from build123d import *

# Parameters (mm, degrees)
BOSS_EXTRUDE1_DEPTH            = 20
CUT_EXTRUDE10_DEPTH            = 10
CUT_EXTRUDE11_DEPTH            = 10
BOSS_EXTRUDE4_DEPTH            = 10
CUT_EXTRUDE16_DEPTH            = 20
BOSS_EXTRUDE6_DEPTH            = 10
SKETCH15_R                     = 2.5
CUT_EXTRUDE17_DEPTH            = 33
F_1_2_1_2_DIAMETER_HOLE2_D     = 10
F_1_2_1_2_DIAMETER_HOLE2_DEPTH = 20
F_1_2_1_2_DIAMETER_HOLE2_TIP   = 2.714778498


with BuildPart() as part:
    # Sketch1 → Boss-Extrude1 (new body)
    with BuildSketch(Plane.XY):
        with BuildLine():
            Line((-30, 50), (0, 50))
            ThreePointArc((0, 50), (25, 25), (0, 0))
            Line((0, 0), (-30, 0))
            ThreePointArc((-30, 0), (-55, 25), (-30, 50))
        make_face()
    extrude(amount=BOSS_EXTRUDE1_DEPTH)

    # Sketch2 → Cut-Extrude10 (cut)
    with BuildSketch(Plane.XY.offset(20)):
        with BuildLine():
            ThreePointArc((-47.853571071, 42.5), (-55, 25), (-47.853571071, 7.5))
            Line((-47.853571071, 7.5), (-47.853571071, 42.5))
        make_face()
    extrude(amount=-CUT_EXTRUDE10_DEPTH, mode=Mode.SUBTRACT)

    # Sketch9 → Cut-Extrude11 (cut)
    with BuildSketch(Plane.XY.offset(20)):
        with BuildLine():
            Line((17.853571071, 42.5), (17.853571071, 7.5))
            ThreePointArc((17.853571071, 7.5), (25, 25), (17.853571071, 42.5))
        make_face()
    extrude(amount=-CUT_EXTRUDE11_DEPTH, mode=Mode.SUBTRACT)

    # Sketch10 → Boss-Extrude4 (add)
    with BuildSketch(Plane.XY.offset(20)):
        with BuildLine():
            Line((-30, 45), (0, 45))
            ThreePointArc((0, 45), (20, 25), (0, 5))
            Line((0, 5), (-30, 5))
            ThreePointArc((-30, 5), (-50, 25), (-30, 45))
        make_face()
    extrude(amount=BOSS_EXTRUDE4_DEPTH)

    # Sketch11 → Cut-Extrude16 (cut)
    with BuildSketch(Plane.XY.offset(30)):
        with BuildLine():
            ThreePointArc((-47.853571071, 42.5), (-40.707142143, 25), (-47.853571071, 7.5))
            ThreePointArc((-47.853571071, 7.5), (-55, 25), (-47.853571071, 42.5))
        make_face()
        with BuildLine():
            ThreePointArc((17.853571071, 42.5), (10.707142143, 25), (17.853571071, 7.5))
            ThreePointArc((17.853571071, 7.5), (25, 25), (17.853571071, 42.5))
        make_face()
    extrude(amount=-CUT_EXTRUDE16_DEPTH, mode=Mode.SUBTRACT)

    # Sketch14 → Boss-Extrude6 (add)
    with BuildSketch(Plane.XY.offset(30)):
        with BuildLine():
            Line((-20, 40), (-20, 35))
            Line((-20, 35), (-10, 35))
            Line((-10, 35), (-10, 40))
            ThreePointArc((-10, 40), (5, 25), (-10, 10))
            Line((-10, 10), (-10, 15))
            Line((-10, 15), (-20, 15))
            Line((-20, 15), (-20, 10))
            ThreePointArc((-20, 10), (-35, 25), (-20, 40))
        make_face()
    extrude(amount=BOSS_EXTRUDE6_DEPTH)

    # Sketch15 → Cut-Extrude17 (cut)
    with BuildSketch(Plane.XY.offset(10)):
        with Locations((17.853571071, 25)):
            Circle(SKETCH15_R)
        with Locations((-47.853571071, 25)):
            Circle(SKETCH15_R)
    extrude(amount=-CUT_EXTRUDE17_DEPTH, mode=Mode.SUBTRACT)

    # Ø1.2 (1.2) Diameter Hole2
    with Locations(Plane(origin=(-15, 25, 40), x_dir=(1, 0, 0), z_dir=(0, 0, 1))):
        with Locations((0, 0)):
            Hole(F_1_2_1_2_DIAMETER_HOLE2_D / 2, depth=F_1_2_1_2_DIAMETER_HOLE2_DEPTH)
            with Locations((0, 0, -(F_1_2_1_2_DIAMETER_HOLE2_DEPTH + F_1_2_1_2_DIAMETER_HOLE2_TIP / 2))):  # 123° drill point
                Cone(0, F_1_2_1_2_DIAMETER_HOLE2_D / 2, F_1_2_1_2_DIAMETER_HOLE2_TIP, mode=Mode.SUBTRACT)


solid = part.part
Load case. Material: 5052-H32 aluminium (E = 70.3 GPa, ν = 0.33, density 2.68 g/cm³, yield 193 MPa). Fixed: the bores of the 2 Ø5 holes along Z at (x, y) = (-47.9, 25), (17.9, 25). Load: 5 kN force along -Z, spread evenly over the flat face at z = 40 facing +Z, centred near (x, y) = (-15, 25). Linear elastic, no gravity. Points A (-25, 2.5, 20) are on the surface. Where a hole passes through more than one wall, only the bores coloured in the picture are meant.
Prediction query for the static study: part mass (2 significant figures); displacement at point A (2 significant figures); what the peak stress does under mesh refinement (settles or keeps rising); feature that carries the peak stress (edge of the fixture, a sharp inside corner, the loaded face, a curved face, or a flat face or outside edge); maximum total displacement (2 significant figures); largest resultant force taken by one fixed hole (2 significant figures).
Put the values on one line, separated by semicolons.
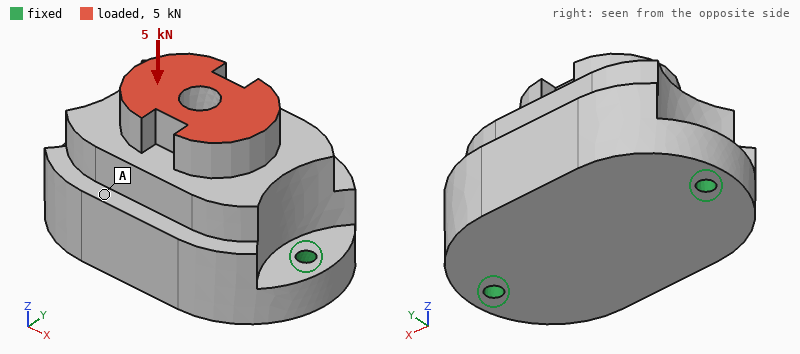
240 g; 8.8 µm; keeps rising; edge of the fixture; 9.9 µm; 2.7 kN
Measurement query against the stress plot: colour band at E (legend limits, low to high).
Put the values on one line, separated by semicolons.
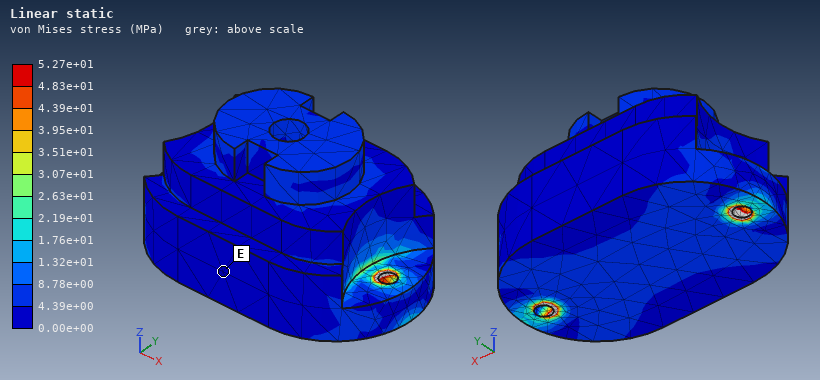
0.00e+00 to 4.39e+00 MPa
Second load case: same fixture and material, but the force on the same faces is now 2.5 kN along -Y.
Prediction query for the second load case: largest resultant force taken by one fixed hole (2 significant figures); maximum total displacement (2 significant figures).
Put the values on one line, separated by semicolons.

1.3 kN; 85 µm
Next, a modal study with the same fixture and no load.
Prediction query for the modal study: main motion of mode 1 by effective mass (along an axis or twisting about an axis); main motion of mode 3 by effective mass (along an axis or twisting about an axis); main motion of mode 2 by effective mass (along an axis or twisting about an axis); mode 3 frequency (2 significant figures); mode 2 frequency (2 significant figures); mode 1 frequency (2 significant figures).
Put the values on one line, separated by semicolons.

along Y; along X; along Z; 11 kHz; 8300 Hz; 3400 Hz
